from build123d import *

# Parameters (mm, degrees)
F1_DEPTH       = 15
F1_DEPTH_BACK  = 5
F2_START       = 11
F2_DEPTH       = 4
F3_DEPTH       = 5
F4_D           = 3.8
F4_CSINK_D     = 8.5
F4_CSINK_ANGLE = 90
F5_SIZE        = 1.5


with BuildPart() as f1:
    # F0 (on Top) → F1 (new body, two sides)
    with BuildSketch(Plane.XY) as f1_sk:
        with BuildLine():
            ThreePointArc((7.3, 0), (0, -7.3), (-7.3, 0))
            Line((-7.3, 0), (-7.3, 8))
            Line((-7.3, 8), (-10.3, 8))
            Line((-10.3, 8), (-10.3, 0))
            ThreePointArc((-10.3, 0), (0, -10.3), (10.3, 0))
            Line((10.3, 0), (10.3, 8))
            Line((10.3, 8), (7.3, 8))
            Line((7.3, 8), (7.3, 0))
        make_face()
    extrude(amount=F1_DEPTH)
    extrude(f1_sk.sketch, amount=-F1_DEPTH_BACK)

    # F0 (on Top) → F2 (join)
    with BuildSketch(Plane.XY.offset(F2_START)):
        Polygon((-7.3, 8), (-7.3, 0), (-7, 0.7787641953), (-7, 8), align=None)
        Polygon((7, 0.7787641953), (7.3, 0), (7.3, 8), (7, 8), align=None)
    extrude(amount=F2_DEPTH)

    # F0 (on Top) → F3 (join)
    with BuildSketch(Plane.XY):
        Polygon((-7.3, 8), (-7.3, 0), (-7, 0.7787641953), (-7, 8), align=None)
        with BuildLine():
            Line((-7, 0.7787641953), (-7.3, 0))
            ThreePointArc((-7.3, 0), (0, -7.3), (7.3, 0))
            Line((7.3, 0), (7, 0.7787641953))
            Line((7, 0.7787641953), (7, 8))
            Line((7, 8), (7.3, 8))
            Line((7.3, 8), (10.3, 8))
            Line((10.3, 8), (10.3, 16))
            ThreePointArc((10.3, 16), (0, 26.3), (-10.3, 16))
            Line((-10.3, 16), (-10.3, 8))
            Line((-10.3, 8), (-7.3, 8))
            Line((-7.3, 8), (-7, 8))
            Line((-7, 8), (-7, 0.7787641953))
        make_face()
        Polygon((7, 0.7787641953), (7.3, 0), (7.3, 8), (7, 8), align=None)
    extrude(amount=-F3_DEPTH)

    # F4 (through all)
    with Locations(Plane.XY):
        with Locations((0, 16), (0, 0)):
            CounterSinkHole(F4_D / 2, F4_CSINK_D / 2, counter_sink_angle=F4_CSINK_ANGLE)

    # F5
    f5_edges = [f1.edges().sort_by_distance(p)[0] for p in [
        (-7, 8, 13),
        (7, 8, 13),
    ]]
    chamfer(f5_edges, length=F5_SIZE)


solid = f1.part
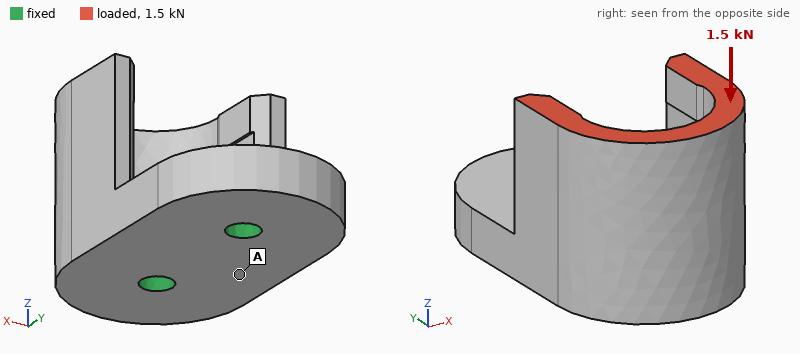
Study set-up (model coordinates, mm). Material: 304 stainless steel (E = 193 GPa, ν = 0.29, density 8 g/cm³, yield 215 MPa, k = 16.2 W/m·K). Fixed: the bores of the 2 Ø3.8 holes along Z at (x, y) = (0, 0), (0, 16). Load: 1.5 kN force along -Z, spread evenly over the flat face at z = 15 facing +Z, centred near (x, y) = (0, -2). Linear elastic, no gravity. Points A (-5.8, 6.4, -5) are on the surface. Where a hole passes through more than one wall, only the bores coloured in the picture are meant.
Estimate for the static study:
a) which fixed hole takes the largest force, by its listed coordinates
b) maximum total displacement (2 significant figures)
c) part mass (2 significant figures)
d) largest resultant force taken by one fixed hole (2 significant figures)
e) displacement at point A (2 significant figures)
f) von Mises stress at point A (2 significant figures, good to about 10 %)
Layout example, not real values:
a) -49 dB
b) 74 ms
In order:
a) (0, 0)
b) 8.3 µm
c) 41 g
d) 1.5 kN
e) 1.3 µm
f) 14 MPa
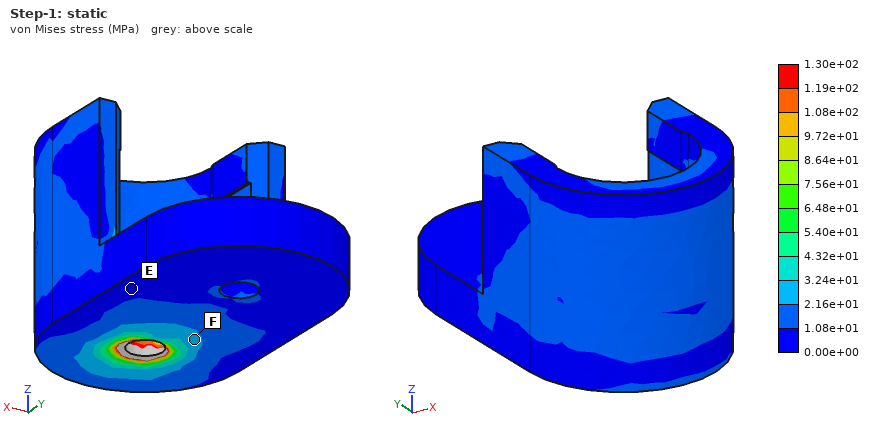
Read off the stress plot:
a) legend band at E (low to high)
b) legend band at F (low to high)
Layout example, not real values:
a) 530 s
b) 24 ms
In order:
a) 0.00e+00 to 1.08e+01 MPa
b) 2.16e+01 to 3.24e+01 MPa
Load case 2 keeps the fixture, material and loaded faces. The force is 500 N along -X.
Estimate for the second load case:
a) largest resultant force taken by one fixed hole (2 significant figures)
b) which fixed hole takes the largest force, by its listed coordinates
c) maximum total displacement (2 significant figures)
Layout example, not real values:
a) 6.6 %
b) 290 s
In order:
a) 490 N
b) (0, 0)
c) 47 µm
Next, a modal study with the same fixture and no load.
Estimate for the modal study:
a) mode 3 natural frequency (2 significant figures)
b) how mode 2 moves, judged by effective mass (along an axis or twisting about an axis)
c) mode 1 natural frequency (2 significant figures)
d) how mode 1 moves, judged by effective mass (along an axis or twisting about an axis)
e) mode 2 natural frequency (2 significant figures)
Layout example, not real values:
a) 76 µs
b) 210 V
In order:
a) 14 kHz
b) along Y
c) 6700 Hz
d) along X
e) 11 kHz
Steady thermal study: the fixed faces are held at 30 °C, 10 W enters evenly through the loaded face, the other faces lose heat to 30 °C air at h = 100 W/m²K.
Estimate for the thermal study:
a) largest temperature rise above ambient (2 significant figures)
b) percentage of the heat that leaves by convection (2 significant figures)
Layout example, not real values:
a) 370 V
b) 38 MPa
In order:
a) 65 K
b) 63 %
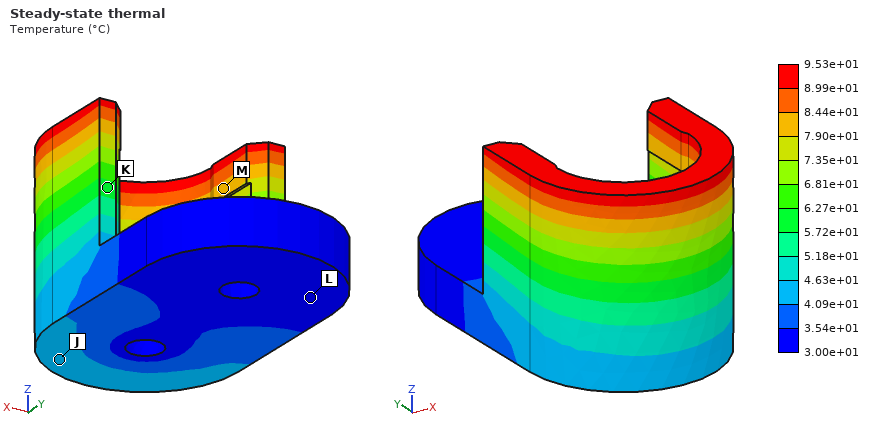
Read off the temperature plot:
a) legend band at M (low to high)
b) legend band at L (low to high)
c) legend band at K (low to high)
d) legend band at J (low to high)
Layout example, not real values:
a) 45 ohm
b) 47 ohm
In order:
a) 7.90e+01 to 8.44e+01 °C
b) 3.00e+01 to 3.54e+01 °C
c) 5.72e+01 to 6.27e+01 °C
d) 4.09e+01 to 4.63e+01 °C
